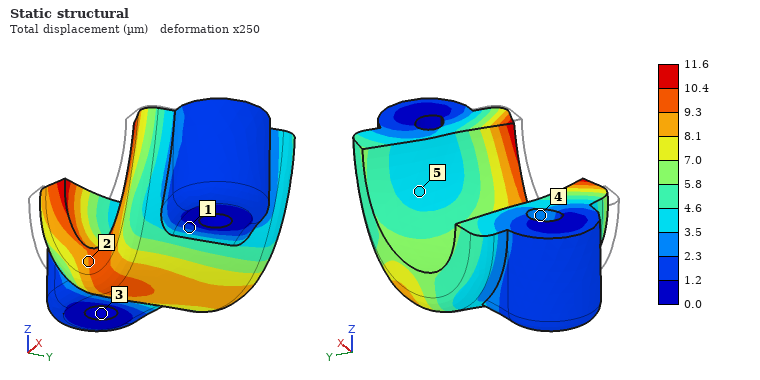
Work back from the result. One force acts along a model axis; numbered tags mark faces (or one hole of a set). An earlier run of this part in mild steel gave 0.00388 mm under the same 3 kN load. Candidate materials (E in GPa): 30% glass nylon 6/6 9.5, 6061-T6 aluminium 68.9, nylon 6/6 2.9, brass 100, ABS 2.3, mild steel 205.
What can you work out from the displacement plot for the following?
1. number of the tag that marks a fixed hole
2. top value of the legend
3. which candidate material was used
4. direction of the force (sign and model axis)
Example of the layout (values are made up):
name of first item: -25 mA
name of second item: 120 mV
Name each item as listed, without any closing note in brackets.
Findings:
number of the tag that marks a fixed hole: 3
top value of the legend: 11.6 µm
which candidate material was used: 6061-T6 aluminium
direction of the force: +Y
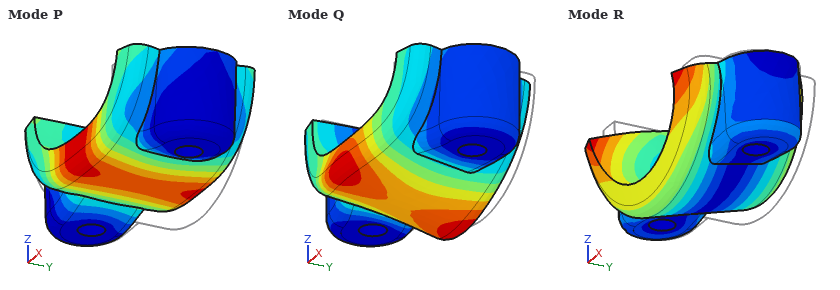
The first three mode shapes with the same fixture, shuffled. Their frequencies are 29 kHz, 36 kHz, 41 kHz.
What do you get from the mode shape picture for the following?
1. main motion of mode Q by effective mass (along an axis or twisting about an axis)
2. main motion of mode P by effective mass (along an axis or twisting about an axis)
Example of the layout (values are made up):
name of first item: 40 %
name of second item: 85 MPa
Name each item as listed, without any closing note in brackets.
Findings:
main motion of mode Q by effective mass: along Y
main motion of mode P by effective mass: along Z
